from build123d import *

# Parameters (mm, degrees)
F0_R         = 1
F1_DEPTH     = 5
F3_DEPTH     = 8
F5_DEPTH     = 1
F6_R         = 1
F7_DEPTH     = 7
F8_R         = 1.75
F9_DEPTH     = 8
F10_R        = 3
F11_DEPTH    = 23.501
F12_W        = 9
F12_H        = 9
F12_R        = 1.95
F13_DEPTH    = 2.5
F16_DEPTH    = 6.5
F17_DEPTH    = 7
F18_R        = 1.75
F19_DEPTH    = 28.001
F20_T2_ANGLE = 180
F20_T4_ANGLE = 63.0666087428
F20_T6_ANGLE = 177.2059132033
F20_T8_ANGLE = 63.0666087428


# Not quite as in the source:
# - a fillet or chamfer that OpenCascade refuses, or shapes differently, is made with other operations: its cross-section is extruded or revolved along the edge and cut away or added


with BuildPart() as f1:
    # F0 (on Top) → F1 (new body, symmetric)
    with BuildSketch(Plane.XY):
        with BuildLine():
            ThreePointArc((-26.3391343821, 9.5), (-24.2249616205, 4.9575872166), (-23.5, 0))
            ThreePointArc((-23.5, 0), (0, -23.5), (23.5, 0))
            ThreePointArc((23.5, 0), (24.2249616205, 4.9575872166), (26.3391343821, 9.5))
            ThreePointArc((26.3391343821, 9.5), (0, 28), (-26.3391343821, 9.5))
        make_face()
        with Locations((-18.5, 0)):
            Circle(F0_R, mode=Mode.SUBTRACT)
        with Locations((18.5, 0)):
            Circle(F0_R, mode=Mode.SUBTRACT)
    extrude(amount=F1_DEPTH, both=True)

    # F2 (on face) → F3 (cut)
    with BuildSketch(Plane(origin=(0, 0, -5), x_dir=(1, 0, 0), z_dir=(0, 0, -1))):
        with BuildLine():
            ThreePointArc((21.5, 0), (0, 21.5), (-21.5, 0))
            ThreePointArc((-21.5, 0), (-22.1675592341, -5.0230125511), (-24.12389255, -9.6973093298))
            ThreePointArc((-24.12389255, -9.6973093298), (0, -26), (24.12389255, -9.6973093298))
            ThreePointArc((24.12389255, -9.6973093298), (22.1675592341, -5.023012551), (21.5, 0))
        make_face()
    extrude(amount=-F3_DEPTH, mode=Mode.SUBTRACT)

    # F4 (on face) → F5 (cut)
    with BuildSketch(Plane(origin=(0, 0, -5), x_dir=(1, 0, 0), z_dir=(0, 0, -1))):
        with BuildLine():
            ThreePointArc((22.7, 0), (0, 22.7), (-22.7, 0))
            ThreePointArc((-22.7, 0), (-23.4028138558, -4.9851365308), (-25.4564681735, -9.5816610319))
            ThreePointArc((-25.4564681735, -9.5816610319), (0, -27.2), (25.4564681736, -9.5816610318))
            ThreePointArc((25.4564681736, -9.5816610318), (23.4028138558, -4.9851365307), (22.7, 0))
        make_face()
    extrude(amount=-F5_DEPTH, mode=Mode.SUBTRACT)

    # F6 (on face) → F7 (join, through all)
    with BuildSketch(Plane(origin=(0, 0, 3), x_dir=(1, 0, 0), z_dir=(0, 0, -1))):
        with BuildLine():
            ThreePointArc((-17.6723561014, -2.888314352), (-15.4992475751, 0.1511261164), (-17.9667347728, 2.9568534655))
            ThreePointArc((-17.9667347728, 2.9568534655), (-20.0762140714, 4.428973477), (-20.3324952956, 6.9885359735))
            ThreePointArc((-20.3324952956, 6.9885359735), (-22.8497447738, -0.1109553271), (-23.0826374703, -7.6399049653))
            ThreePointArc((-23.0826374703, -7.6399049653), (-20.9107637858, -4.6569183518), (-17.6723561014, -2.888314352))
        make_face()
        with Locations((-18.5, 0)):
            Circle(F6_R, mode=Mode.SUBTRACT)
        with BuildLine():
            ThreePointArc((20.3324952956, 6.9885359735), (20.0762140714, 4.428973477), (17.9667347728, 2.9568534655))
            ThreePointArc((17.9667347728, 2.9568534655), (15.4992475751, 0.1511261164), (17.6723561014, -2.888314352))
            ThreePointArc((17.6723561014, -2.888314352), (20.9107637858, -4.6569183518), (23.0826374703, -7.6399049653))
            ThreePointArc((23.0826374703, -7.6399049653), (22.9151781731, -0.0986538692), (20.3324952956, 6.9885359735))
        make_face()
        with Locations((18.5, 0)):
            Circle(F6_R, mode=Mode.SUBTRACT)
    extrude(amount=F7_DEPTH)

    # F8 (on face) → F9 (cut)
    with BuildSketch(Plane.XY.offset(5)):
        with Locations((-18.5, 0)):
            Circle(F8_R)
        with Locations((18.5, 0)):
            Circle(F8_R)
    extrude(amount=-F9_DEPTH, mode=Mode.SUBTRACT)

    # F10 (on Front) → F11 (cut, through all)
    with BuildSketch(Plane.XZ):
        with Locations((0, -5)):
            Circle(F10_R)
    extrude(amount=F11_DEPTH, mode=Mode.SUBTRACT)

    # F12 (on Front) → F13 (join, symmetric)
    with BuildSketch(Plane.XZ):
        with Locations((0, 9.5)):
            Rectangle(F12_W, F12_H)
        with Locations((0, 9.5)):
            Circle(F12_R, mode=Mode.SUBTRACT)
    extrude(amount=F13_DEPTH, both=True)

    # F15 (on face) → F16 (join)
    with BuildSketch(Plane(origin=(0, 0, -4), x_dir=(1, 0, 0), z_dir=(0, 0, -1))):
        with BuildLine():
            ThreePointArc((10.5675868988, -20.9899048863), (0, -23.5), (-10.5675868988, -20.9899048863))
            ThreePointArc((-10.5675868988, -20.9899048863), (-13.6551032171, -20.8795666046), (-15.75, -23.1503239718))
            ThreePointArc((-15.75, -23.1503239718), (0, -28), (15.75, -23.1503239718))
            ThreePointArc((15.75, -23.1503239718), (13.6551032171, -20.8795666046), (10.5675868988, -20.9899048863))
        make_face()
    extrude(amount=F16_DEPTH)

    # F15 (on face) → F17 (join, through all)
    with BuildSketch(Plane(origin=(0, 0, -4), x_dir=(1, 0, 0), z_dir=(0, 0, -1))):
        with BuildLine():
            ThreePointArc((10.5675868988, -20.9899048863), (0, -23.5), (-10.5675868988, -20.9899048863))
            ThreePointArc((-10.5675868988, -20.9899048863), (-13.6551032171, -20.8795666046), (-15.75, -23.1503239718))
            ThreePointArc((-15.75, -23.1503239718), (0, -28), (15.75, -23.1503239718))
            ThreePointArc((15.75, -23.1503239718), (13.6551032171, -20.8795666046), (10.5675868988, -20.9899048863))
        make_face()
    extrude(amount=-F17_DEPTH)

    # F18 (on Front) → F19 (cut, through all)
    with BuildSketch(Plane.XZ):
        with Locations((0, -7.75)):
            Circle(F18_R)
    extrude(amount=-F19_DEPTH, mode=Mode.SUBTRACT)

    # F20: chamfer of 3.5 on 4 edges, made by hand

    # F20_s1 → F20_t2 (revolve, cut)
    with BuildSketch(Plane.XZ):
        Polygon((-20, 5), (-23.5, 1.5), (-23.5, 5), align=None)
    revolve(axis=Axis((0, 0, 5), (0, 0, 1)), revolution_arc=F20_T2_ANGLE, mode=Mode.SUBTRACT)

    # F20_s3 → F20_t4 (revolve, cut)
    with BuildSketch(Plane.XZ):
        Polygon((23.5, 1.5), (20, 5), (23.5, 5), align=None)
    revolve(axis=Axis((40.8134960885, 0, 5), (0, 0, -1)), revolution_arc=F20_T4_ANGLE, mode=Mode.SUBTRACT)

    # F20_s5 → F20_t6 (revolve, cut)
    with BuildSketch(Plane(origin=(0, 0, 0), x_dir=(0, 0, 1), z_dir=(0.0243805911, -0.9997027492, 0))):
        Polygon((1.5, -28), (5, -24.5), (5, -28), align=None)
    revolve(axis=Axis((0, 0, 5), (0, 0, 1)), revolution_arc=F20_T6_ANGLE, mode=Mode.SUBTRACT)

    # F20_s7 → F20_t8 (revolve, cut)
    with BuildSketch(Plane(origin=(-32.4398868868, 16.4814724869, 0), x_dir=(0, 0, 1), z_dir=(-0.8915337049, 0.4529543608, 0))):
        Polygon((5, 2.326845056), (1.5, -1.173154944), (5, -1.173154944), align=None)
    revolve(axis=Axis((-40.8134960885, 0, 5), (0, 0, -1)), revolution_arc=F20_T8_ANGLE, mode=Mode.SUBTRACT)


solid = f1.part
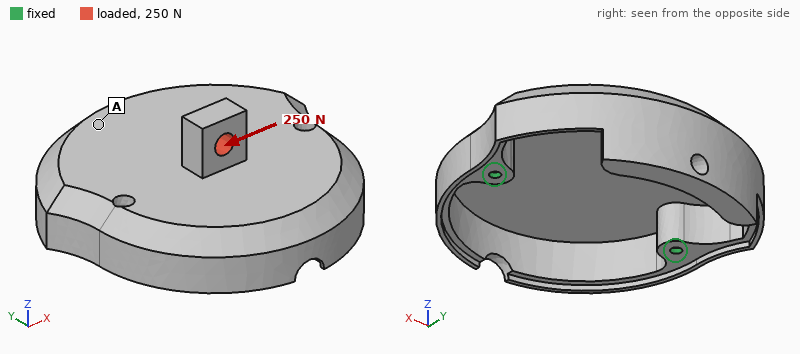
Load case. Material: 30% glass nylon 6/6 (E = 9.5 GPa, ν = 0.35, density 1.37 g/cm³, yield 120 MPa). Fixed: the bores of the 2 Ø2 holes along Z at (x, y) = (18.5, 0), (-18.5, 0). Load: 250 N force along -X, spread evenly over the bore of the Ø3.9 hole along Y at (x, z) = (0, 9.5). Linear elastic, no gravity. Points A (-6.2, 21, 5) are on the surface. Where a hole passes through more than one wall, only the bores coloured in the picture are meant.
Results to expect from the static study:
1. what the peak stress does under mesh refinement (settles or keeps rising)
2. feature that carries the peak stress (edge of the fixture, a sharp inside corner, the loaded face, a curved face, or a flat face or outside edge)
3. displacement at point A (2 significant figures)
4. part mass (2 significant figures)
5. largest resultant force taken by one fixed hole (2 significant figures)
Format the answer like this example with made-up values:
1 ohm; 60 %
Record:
keeps rising; edge of the fixture; 0.093 mm; 10 g; 150 N
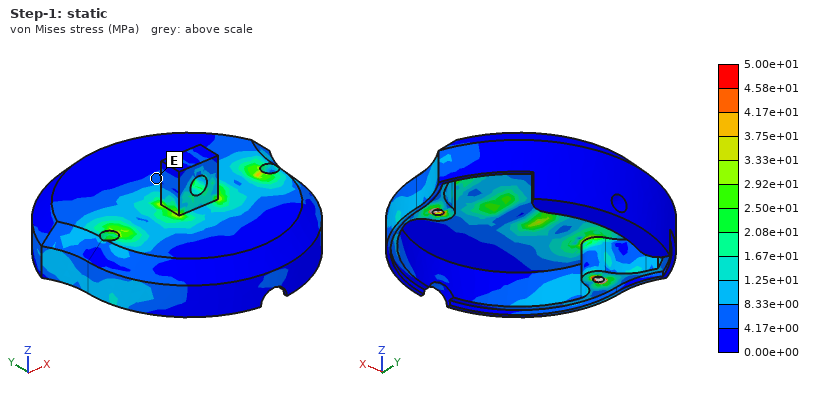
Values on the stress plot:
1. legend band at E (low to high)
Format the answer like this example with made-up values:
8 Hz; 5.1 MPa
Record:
4.17e+00 to 8.33e+00 MPa
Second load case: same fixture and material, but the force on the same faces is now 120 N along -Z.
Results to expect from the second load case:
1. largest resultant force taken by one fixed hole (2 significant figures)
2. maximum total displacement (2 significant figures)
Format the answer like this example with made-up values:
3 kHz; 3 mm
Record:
71 N; 0.12 mm
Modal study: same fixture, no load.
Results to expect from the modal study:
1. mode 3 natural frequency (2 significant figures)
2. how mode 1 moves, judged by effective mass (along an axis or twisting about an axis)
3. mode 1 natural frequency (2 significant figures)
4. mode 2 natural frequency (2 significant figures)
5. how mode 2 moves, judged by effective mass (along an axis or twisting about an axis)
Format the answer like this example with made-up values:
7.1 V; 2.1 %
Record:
2000 Hz; along Z; 580 Hz; 1800 Hz; along X
